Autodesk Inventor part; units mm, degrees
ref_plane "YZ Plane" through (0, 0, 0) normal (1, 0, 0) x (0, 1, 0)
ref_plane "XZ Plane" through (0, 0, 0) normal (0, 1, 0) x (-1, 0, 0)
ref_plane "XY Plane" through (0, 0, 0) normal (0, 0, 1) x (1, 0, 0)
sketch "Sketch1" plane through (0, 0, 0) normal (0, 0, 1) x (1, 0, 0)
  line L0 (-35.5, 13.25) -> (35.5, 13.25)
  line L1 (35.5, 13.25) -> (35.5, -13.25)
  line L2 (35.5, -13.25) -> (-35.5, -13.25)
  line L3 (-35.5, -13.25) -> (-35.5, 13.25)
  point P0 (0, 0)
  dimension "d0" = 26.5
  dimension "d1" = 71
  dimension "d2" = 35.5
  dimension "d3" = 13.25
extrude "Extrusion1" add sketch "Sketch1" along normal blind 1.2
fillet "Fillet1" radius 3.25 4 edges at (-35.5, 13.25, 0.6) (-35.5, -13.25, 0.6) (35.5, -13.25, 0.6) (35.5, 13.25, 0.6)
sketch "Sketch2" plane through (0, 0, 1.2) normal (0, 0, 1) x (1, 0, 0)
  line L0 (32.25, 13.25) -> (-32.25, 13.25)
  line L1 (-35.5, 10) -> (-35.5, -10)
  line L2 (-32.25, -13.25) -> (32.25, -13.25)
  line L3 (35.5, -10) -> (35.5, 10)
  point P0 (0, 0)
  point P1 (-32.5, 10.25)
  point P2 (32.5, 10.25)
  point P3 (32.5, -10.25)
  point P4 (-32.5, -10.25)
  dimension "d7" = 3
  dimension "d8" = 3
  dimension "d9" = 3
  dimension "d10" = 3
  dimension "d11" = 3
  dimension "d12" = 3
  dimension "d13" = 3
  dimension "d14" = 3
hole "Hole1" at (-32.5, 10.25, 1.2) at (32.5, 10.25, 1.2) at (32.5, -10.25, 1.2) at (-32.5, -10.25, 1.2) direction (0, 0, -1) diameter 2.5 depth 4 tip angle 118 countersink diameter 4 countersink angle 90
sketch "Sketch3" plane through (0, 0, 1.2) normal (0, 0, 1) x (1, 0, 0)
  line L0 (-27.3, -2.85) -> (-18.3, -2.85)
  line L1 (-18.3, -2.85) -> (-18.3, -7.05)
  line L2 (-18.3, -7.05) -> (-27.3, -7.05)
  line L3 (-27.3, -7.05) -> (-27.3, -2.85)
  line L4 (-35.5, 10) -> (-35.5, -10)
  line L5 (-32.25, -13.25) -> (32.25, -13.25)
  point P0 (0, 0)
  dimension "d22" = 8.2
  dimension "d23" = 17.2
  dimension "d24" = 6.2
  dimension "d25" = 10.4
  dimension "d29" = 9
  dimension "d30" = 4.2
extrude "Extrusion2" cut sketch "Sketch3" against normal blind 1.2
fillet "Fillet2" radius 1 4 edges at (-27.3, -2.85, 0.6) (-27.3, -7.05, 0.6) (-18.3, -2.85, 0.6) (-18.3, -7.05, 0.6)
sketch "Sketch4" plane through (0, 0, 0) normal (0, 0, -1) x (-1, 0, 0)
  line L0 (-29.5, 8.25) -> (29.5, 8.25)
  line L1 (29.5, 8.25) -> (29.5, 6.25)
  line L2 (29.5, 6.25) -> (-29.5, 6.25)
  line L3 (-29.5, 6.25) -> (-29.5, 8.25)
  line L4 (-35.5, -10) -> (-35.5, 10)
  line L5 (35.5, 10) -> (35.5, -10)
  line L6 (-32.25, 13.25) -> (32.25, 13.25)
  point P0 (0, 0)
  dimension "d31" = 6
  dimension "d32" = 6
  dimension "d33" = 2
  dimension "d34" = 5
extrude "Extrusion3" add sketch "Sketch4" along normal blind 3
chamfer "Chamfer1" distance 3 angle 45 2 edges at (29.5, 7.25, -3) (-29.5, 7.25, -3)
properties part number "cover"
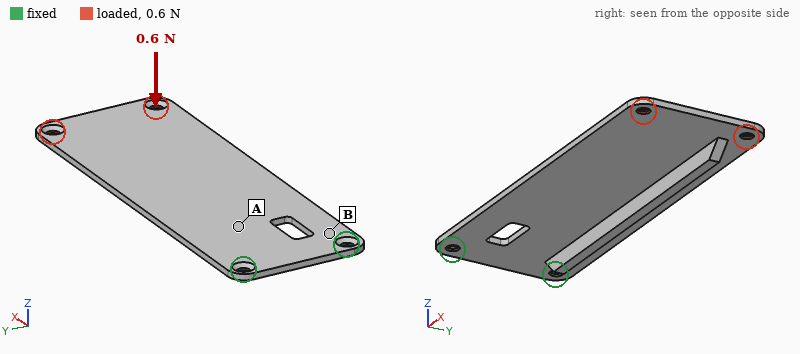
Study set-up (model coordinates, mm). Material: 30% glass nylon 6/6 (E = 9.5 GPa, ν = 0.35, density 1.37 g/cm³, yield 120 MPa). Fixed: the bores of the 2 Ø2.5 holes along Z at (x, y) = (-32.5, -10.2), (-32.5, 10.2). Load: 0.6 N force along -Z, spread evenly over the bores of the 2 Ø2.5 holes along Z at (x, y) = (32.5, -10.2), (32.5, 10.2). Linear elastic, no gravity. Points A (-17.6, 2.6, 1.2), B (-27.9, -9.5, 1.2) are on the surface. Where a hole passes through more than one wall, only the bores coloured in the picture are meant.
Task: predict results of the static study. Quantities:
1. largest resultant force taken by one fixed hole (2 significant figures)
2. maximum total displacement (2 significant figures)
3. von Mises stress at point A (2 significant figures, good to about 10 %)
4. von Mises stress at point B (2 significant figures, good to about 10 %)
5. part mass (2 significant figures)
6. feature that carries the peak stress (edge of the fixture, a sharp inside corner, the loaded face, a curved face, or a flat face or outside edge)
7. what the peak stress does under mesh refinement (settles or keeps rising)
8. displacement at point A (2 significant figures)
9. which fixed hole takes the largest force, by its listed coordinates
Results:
0.50 N
0.86 mm
1.6 MPa
3.7 MPa
3.4 g
edge of the fixture
keeps rising
0.13 mm
(-32.5, -10.2)
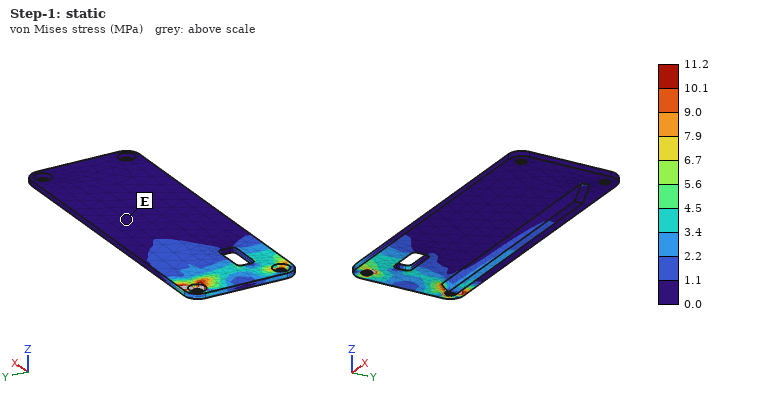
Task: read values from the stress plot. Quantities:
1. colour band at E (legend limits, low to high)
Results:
0.0 to 1.1 MPa
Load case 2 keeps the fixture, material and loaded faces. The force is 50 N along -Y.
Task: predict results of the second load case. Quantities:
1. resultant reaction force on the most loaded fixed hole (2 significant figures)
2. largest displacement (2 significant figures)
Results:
160 N
0.88 mm
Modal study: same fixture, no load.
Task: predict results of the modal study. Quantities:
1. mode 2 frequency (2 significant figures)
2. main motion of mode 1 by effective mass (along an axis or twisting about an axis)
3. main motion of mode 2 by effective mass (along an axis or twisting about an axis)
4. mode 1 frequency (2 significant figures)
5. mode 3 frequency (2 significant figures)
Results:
660 Hz
along Z
twisting about X
130 Hz
1200 Hz
